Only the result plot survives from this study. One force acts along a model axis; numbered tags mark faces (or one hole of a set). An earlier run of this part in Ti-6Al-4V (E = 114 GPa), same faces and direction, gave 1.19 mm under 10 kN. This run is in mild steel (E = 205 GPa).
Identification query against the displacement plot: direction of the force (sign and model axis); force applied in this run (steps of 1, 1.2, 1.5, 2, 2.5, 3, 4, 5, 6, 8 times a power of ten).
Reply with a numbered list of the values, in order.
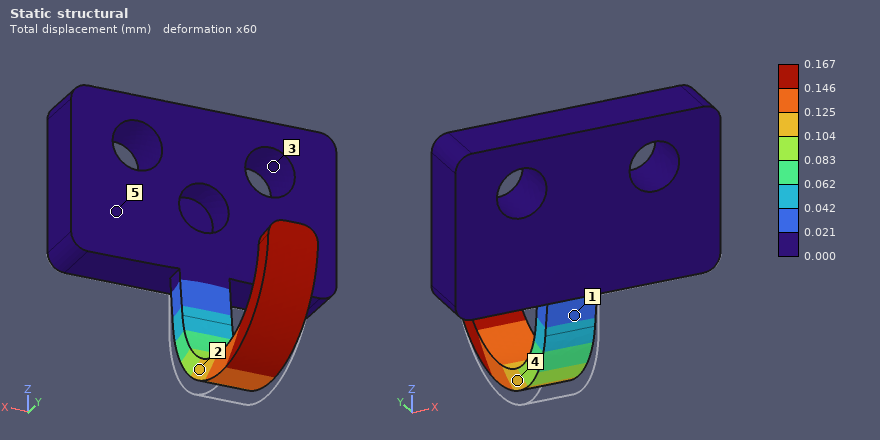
1. +Y
2. 2.5 kN
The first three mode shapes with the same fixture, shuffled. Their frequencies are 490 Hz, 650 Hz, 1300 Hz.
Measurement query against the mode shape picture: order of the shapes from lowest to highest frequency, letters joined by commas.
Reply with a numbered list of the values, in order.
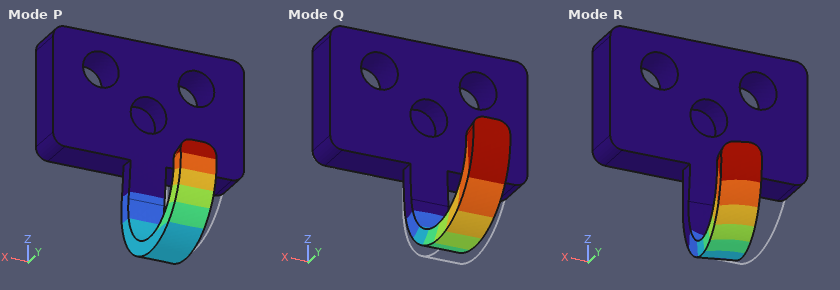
1. Q, R, P
